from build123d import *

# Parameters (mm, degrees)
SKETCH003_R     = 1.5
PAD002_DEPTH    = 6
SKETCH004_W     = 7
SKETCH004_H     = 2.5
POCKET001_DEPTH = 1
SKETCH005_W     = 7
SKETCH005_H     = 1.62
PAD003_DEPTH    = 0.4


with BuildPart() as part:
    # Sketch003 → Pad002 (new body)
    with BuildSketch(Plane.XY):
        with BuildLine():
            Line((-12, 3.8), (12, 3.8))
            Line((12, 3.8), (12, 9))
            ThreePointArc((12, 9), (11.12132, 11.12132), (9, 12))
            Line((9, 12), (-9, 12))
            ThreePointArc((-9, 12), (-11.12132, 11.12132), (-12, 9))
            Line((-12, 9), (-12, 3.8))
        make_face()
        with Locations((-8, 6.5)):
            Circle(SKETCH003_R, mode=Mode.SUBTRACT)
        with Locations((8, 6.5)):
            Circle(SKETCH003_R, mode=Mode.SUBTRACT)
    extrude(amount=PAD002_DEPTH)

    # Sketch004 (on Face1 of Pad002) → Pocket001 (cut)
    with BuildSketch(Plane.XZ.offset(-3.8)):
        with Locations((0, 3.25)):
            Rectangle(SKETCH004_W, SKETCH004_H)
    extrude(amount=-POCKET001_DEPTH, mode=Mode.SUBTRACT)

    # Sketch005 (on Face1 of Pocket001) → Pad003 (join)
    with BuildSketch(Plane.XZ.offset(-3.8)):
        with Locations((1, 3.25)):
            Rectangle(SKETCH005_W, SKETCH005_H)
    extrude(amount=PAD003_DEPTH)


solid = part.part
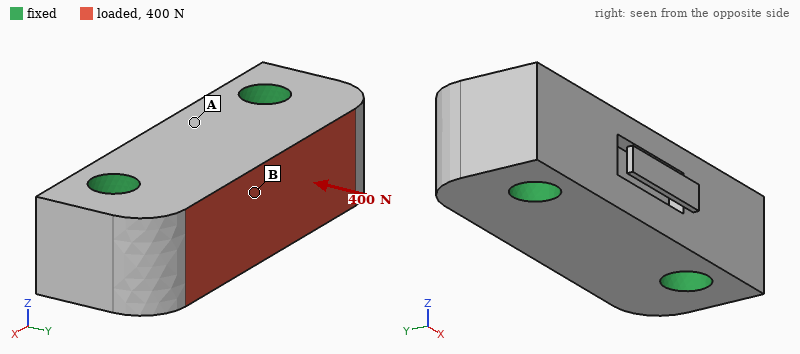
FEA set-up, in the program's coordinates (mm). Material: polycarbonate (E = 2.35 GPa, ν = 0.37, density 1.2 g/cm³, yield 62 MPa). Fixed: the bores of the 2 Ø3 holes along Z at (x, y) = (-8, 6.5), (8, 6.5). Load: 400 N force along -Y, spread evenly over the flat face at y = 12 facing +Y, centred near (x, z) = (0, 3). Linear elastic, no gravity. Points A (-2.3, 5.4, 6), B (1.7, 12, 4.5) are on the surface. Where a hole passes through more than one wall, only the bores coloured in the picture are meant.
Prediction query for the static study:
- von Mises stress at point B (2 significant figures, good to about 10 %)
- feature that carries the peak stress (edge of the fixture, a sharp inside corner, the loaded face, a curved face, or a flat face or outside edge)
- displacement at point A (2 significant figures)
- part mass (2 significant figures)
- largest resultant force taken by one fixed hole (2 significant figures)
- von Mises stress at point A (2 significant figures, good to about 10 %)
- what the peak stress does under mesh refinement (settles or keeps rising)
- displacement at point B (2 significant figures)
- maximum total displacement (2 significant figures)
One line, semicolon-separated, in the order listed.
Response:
5.7 MPa; edge of the fixture; 22 µm; 1.3 g; 210 N; 2.4 MPa; keeps rising; 26 µm; 42 µm
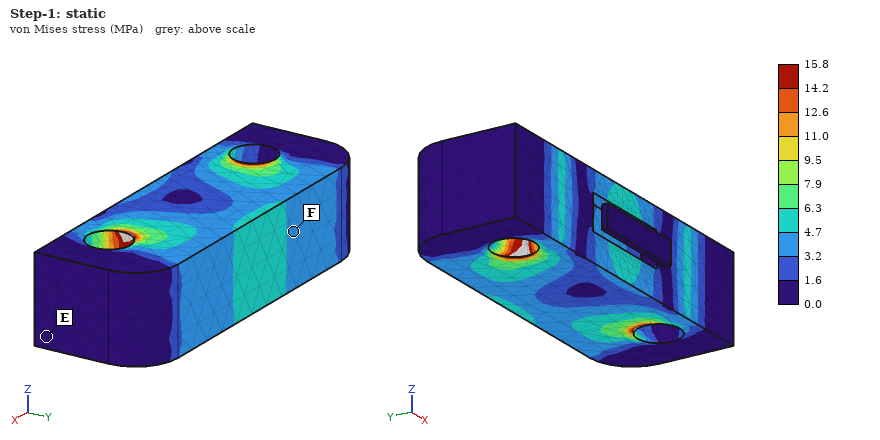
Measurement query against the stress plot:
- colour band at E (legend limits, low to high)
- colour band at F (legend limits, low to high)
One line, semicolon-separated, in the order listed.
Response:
0.0 to 1.6 MPa; 3.2 to 4.7 MPa
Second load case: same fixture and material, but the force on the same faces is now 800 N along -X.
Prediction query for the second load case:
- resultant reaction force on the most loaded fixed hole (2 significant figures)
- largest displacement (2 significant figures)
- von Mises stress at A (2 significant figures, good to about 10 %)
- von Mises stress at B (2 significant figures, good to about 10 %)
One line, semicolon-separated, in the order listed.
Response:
450 N; 47 µm; 3.3 MPa; 13 MPa
